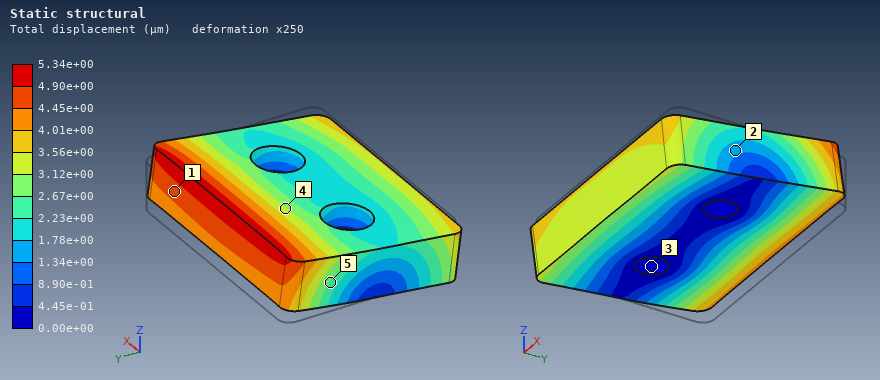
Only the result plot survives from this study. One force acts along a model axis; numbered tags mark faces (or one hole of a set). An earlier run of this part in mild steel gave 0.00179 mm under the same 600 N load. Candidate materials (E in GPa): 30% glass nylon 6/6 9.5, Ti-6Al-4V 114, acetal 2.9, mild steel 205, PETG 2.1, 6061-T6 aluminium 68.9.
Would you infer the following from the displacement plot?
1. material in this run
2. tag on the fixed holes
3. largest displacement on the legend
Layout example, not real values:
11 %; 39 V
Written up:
6061-T6 aluminium; 3; 5.34e+00 µm
